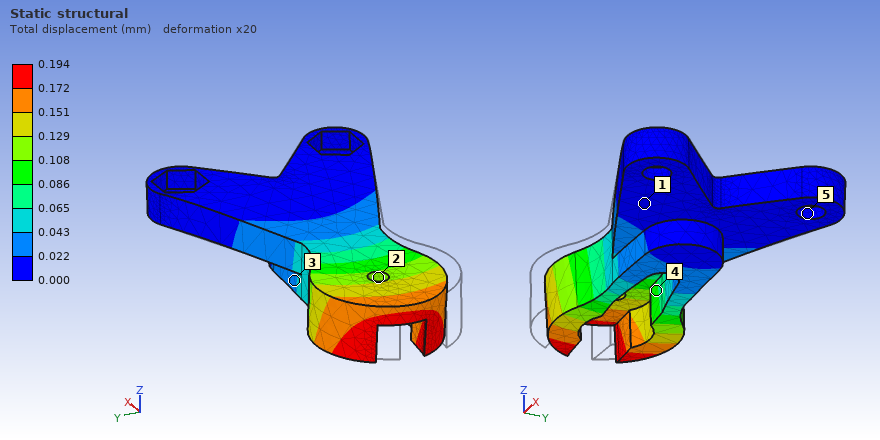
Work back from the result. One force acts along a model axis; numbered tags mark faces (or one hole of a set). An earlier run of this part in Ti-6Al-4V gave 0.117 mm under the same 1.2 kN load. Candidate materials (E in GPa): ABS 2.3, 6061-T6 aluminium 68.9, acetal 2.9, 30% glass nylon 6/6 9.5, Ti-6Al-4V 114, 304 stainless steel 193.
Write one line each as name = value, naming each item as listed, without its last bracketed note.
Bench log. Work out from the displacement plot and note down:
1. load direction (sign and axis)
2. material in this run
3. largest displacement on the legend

load direction = +Y
material in this run = 6061-T6 aluminium
largest displacement on the legend = 0.194 mm
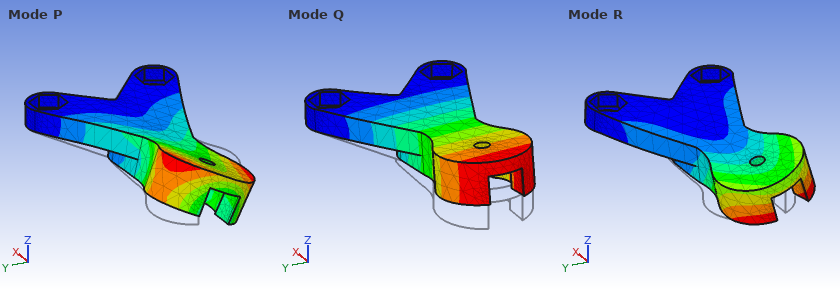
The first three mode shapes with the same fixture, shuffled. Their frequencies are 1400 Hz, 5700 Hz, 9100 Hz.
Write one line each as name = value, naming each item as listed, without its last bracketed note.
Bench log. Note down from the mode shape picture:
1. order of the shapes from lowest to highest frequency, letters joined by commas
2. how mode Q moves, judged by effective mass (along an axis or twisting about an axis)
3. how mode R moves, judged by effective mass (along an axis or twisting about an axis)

order of the shapes from lowest to highest frequency, letters joined by commas = Q, R, P
how mode Q moves, judged by effective mass = along Z
how mode R moves, judged by effective mass = along Y
